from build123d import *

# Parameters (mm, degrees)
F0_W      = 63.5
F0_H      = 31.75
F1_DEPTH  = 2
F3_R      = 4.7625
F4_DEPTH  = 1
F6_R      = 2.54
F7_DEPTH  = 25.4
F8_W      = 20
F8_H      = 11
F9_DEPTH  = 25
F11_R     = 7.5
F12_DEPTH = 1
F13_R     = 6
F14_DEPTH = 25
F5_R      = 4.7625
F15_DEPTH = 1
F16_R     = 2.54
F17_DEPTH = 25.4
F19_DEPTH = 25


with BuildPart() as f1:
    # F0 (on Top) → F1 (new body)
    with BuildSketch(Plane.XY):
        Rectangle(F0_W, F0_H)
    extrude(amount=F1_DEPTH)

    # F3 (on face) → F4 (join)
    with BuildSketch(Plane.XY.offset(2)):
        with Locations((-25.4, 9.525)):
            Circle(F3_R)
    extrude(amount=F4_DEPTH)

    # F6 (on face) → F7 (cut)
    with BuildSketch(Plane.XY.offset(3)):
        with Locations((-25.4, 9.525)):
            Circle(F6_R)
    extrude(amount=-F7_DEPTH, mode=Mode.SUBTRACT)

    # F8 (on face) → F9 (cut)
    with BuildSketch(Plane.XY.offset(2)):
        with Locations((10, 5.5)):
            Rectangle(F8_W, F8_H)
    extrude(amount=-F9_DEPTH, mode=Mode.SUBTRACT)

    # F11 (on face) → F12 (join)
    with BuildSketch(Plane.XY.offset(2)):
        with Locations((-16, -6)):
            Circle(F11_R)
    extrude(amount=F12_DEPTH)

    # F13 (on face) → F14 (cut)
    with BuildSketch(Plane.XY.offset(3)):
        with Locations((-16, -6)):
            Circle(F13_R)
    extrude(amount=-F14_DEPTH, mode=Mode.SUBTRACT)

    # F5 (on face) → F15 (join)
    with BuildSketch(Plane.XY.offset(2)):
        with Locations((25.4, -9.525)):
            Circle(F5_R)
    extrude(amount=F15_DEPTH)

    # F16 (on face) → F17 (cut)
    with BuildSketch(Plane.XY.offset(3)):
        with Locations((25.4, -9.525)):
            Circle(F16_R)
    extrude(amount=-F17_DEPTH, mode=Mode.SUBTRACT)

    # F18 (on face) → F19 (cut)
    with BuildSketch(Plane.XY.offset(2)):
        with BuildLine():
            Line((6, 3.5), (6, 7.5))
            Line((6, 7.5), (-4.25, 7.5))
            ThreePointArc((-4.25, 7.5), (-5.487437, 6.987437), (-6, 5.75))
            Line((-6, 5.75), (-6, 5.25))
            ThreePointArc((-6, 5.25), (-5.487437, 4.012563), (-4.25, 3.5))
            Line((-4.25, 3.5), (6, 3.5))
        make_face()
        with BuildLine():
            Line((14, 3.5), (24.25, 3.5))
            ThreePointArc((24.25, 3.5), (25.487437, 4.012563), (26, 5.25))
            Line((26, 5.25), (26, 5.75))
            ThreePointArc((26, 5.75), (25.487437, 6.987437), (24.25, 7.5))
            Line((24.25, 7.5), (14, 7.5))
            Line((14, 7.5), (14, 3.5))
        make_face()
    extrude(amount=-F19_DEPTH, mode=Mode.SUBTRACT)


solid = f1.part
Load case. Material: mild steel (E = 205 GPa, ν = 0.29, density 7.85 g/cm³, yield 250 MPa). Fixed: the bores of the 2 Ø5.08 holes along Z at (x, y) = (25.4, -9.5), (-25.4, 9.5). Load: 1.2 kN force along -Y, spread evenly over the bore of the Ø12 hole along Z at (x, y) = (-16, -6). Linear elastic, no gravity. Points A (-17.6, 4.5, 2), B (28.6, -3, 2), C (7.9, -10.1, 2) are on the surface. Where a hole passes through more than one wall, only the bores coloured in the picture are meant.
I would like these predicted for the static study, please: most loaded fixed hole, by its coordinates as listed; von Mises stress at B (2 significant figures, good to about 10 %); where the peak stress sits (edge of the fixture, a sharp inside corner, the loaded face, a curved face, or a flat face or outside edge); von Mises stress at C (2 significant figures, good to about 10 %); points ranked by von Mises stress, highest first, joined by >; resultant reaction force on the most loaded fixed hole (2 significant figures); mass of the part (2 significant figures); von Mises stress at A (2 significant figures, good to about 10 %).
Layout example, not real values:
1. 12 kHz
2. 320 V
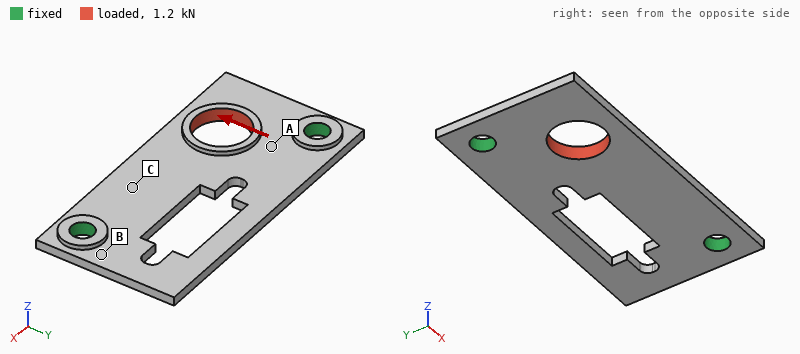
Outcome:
1. (-25.4, 9.5)
2. 9.9 MPa
3. edge of the fixture
4. 22 MPa
5. A > C > B
6. 1.1 kN
7. 26 g
8. 50 MPa
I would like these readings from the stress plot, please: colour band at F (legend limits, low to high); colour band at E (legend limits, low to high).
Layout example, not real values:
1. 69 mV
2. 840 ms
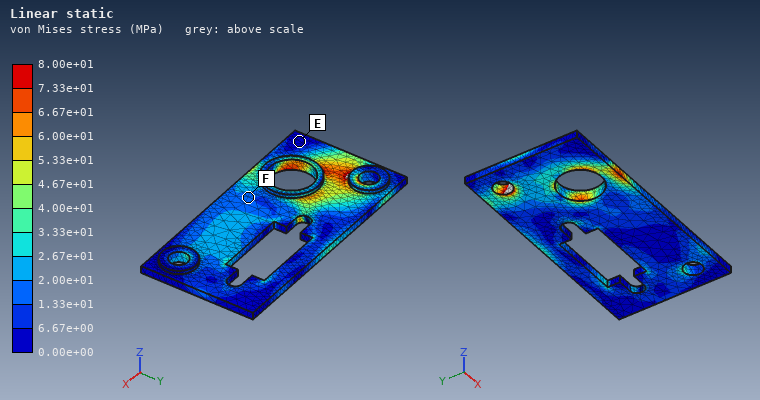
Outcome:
1. 1.33e+01 to 2.00e+01 MPa
2. 0.00e+00 to 6.67e+00 MPa
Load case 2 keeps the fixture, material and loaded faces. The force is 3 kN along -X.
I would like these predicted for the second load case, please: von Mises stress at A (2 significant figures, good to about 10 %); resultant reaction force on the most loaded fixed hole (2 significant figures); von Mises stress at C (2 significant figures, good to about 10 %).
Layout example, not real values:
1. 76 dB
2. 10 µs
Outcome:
1. 77 MPa
2. 1.5 kN
3. 68 MPa
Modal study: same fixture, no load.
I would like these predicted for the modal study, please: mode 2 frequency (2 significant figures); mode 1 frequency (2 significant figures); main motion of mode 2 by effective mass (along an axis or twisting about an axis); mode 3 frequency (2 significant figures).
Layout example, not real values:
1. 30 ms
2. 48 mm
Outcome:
1. 3100 Hz
2. 2800 Hz
3. along Z
4. 4800 Hz
